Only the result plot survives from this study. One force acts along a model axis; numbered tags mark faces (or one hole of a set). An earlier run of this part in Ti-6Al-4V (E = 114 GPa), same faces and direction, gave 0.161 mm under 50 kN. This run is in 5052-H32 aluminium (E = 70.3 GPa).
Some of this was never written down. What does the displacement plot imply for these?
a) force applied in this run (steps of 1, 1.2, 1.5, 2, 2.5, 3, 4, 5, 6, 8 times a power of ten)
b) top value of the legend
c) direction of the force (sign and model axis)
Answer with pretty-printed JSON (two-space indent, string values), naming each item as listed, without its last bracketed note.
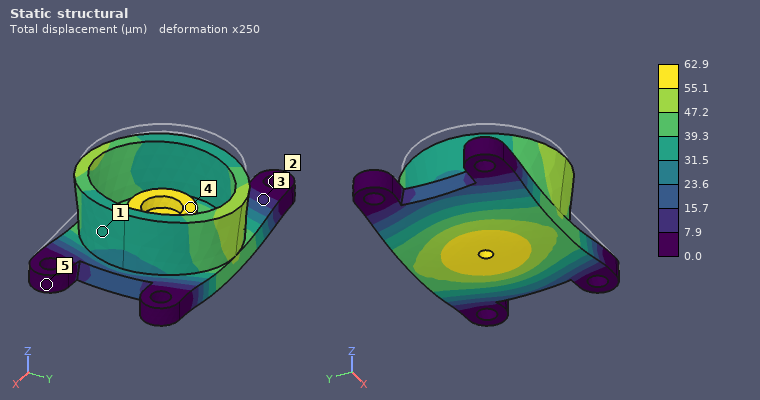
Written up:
{
  "force applied in this run": "12 kN",
  "top value of the legend": "62.9 µm",
  "direction of the force": "-Z"
}
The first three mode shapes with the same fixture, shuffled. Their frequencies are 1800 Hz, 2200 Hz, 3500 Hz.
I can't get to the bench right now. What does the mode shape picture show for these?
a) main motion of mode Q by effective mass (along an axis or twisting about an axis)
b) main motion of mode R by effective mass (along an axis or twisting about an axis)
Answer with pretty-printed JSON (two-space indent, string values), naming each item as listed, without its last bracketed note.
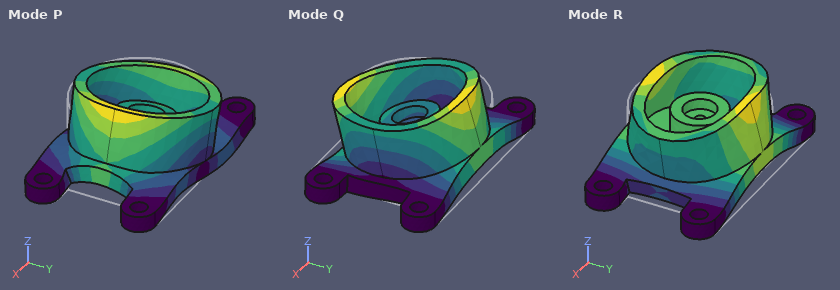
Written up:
{
  "main motion of mode Q by effective mass": "along Y",
  "main motion of mode R by effective mass": "along Z"
}
